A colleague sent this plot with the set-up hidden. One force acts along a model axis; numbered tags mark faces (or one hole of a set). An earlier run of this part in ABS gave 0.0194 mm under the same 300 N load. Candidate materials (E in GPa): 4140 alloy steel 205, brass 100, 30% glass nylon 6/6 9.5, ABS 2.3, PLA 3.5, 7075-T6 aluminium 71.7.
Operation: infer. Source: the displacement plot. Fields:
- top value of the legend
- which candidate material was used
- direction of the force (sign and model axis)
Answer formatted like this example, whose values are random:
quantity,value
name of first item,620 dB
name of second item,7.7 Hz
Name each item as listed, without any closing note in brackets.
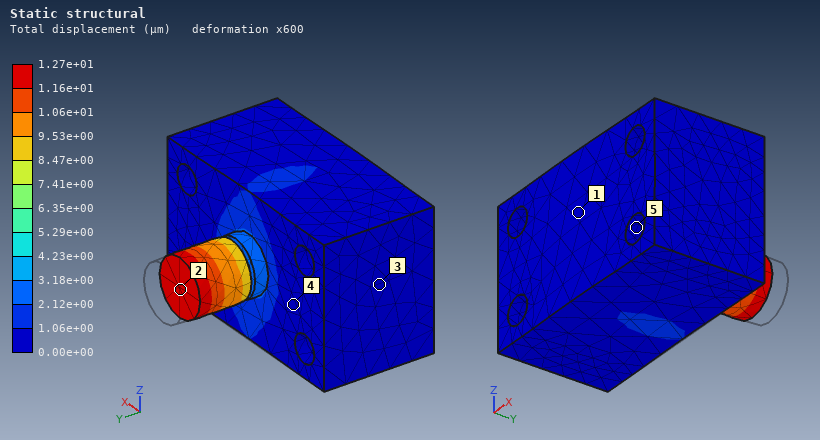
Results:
quantity,value
top value of the legend,1.27e+01 µm
which candidate material was used,PLA
direction of the force,-Y
